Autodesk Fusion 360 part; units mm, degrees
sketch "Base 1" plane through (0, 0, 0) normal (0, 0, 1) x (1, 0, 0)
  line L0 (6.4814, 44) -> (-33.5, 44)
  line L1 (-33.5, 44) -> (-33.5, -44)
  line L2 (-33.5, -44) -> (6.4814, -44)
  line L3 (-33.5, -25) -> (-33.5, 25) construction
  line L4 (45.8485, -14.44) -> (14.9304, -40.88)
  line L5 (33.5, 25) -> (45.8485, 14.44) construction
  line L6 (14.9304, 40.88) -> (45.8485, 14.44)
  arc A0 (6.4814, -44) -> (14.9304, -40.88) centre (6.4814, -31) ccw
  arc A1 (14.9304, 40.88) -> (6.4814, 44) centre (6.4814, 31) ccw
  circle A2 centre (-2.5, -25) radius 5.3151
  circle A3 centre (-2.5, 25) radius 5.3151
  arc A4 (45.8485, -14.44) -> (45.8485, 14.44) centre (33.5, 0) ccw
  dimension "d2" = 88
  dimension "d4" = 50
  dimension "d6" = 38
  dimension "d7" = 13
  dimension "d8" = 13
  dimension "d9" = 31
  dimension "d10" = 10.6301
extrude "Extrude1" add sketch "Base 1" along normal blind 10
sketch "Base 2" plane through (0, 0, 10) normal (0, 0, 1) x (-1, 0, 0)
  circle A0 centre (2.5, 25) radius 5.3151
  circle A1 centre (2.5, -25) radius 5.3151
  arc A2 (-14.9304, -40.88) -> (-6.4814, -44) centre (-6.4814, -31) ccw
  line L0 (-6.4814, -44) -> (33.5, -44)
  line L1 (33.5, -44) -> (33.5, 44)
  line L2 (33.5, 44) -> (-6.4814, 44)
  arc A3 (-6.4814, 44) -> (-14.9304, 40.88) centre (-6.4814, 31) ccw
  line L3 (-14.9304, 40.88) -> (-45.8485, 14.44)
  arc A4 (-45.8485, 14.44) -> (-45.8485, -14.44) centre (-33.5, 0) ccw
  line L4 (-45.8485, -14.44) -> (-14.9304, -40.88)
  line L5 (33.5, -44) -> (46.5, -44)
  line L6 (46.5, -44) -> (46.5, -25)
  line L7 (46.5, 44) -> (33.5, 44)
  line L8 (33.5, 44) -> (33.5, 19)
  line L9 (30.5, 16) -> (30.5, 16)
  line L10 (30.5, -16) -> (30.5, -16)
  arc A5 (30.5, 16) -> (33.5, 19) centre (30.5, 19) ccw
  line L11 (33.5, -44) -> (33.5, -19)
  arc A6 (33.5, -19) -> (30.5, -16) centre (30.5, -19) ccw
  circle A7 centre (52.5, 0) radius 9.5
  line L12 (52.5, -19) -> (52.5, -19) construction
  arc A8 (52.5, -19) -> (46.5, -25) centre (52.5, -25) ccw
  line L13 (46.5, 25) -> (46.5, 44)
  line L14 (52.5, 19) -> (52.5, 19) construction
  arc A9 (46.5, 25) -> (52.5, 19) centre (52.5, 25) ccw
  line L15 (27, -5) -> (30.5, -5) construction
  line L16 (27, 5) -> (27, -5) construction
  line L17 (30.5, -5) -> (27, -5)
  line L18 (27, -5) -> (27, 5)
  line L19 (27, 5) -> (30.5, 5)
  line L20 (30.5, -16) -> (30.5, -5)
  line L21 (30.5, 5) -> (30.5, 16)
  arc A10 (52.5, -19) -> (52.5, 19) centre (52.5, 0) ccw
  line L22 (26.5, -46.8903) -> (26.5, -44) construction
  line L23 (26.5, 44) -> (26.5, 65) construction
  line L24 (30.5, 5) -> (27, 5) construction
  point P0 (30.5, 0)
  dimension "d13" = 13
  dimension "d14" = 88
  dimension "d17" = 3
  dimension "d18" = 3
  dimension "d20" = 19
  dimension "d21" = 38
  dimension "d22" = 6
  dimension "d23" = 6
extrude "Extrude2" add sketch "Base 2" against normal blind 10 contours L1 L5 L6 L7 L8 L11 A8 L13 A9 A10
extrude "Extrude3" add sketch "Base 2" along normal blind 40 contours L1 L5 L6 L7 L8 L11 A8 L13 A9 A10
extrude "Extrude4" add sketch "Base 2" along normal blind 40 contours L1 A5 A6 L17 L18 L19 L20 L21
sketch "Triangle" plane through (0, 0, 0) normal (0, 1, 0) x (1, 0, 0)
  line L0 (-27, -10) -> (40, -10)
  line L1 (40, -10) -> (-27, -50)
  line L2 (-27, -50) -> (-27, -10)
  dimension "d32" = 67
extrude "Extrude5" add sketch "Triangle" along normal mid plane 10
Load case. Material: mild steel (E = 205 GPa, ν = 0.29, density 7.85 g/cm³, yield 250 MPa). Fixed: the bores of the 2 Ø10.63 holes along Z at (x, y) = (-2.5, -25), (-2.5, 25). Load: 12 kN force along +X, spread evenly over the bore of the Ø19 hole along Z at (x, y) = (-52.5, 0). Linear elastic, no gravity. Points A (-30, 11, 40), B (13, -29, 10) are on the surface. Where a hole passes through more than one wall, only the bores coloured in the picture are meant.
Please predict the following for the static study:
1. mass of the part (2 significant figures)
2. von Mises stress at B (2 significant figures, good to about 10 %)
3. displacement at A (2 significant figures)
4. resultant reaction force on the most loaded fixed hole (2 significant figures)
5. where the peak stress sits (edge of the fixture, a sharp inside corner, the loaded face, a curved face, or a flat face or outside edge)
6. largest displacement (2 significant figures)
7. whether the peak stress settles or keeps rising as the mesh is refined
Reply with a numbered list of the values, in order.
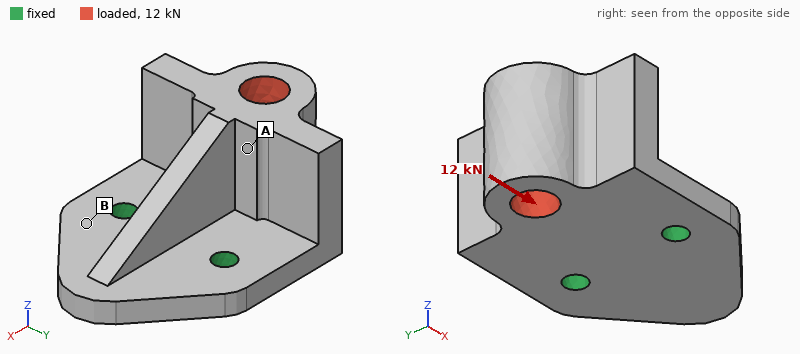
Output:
1. 1.3 kg
2. 44 MPa
3. 0.057 mm
4. 6.0 kN
5. edge of the fixture
6. 0.11 mm
7. keeps rising
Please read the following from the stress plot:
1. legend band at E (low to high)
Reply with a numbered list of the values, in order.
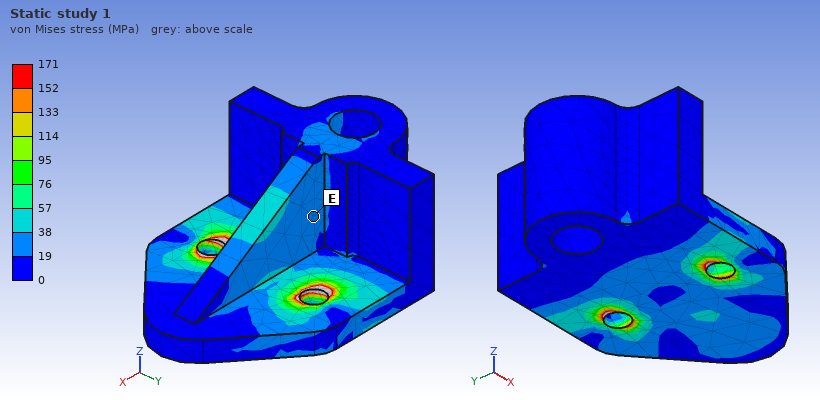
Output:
1. 19 to 38 MPa
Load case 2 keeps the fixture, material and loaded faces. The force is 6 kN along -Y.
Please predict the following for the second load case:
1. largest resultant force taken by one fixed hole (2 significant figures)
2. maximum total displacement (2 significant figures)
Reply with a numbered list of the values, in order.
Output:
1. 6.5 kN
2. 28 µm
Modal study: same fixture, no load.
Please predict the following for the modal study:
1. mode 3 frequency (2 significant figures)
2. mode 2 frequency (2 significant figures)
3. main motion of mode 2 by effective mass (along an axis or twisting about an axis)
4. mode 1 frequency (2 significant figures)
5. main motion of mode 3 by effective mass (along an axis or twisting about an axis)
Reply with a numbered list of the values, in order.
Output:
1. 5600 Hz
2. 2900 Hz
3. along Y
4. 1600 Hz
5. along Z
